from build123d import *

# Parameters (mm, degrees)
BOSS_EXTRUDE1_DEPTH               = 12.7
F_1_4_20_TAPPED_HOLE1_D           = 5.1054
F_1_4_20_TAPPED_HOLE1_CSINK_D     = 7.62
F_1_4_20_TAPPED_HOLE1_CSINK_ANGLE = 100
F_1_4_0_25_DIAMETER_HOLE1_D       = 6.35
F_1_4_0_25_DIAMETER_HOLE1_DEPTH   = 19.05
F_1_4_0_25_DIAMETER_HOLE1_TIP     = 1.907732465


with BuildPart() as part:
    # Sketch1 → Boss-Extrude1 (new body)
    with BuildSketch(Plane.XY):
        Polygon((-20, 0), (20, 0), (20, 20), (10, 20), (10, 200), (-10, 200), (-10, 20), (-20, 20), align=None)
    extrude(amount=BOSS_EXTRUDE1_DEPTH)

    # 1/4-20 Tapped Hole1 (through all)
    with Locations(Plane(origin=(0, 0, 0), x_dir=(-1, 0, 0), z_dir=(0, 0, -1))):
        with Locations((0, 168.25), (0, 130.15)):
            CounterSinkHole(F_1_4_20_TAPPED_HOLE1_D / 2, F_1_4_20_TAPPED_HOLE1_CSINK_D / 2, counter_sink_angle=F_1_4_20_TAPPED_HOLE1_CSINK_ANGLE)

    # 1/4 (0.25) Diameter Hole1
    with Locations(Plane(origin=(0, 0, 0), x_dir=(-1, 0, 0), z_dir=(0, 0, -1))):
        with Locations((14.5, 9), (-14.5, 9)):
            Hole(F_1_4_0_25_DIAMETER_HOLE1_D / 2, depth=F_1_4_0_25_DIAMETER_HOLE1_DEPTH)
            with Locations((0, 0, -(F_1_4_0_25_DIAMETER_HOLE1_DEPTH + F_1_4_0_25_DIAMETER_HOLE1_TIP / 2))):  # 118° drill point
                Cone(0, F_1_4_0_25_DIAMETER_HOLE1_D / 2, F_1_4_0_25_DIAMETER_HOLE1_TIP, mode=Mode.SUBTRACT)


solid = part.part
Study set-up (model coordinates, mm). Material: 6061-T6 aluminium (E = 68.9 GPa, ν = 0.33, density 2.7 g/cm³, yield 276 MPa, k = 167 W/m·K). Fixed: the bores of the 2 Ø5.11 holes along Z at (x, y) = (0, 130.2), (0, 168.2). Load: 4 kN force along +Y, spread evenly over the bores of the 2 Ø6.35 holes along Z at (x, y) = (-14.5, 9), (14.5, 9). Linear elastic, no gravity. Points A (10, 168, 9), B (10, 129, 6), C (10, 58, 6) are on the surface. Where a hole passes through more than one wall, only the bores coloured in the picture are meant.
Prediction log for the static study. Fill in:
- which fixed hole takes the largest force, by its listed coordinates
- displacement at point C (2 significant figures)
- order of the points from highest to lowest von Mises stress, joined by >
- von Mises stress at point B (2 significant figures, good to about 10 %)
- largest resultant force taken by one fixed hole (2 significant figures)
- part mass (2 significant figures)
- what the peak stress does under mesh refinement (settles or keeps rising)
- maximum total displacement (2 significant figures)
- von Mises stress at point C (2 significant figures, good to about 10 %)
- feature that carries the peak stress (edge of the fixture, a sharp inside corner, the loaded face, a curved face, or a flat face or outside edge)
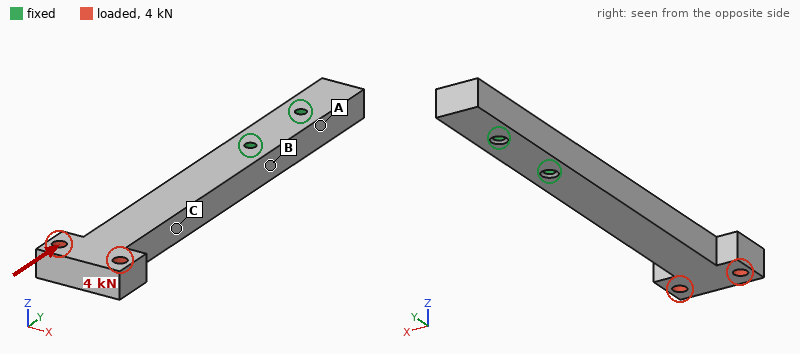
(0, 130.2)
17 µm
C > B > A
8.3 MPa
3.7 kN
150 g
keeps rising
34 µm
16 MPa
edge of the fixture
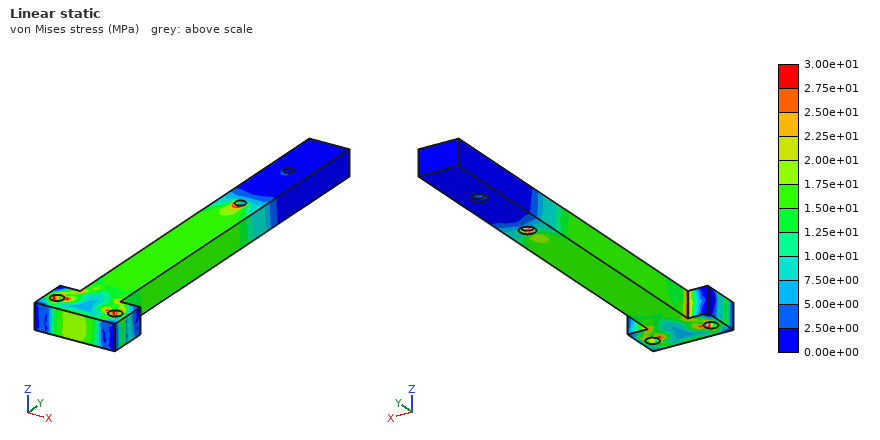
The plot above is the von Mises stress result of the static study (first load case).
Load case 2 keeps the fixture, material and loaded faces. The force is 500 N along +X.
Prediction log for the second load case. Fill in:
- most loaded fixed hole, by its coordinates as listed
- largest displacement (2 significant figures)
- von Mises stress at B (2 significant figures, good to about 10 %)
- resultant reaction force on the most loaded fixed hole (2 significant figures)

(0, 130.2)
0.71 mm
58 MPa
1.5 kN
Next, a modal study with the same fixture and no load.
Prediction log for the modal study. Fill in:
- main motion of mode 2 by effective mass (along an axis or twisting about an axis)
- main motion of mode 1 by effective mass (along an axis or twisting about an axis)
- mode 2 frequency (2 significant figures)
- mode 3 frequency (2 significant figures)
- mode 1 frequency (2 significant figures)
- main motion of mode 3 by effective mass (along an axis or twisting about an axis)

along X
along Z
710 Hz
3200 Hz
500 Hz
twisting about Y
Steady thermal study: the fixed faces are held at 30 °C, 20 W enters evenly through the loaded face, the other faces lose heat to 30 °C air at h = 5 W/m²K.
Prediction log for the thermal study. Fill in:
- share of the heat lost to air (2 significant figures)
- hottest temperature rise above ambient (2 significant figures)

8.0 %
54 K
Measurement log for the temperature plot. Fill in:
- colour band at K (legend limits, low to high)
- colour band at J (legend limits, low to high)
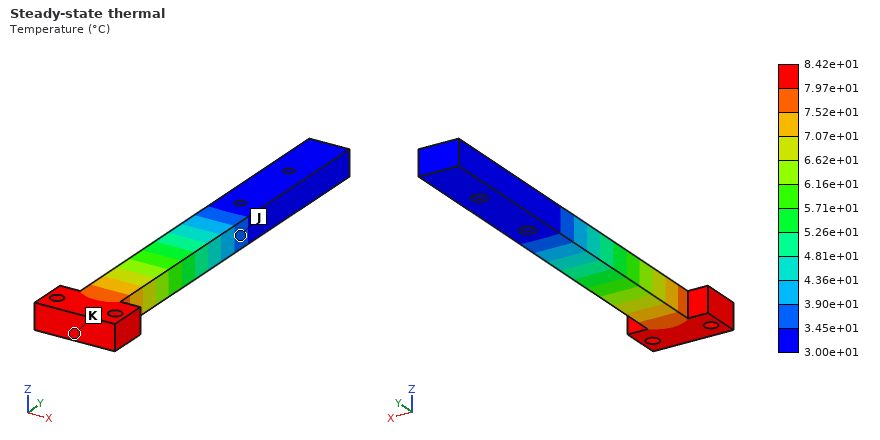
7.97e+01 to 8.42e+01 °C
3.45e+01 to 3.90e+01 °C
